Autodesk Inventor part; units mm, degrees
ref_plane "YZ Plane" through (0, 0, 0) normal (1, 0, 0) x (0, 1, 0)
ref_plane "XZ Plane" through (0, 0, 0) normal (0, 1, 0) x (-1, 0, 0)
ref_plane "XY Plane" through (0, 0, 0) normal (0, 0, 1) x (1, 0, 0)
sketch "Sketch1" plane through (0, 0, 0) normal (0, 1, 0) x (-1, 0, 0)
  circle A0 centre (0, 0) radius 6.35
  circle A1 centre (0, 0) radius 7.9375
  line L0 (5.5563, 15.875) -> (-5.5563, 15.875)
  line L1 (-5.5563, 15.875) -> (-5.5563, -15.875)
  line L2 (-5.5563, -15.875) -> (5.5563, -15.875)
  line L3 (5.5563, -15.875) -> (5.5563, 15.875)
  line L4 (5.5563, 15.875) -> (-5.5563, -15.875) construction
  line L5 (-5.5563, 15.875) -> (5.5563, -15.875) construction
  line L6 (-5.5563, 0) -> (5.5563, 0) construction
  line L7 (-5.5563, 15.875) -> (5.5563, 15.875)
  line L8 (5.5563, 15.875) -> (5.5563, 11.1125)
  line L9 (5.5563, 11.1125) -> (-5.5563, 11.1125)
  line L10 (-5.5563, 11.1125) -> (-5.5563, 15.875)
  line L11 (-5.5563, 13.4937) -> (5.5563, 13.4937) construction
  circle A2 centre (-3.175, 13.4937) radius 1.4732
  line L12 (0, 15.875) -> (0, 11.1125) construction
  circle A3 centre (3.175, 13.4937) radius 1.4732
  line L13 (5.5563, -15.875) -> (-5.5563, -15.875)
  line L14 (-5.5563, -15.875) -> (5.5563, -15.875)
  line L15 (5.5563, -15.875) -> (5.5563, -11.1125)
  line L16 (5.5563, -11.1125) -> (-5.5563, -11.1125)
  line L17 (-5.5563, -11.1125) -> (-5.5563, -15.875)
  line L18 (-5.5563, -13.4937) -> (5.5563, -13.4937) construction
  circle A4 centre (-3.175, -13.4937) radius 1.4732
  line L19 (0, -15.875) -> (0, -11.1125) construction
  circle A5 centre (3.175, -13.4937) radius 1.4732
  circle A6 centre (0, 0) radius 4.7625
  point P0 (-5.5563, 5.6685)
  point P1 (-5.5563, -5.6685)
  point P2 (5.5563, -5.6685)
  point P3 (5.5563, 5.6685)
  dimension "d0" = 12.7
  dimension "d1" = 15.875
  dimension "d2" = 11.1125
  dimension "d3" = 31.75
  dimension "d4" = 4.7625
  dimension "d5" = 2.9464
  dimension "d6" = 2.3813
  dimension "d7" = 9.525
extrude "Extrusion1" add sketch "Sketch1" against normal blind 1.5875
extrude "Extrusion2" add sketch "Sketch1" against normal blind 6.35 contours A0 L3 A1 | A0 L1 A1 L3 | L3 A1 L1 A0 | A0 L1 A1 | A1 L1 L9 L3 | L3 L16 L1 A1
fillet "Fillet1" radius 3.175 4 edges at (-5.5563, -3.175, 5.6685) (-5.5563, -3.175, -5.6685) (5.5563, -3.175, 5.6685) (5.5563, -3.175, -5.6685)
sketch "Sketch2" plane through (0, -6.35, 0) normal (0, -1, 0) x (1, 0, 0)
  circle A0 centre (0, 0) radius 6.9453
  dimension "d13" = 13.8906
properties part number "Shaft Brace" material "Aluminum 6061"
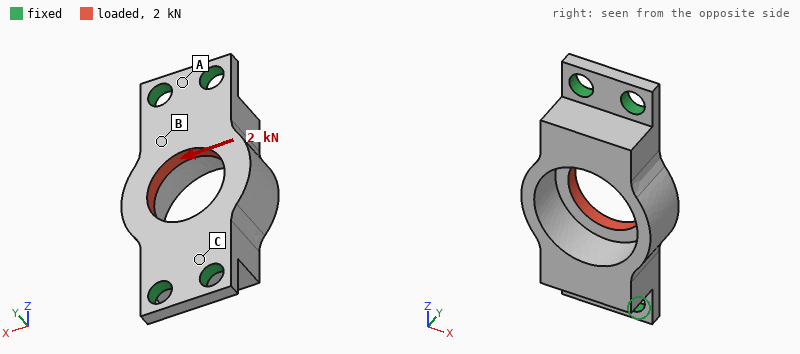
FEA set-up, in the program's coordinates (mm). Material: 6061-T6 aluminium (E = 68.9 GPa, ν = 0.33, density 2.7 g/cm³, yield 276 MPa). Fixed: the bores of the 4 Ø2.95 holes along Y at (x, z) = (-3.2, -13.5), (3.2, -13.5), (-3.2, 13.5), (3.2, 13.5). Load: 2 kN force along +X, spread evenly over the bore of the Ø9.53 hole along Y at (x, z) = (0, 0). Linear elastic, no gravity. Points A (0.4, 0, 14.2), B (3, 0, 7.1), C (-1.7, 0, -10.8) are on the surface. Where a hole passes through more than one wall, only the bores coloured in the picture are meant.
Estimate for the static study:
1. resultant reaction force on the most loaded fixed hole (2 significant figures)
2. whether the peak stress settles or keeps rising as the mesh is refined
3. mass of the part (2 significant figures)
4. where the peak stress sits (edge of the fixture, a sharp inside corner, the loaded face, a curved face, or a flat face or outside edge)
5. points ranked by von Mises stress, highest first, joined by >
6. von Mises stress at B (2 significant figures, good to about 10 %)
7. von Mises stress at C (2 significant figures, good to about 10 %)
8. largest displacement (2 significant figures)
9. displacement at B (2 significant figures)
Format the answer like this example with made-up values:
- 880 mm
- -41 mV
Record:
- 660 N
- keeps rising
- 3.3 g
- edge of the fixture
- C > B > A
- 77 MPa
- 120 MPa
- 29 µm
- 13 µm
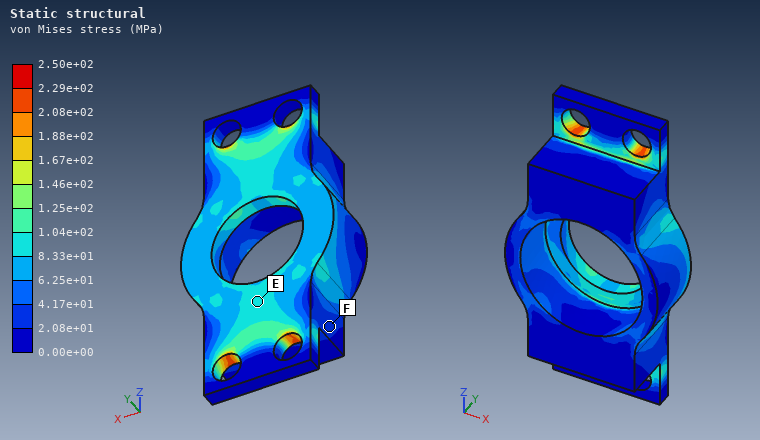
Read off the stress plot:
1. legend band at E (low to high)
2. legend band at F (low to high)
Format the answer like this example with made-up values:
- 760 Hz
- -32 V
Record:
- 8.33e+01 to 1.04e+02 MPa
- 2.08e+01 to 4.17e+01 MPa
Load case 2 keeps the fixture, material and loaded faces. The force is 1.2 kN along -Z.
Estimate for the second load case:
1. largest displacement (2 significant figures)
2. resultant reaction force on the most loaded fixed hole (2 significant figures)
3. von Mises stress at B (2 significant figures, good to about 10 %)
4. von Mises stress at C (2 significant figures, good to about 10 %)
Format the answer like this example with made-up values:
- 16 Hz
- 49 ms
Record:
- 5.8 µm
- 300 N
- 35 MPa
- 25 MPa
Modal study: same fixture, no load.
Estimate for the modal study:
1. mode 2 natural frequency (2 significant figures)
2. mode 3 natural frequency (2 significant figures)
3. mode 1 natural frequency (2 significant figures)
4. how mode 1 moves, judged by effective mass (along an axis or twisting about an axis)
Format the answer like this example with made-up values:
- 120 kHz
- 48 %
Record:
- 23 kHz
- 40 kHz
- 17 kHz
- along Y
